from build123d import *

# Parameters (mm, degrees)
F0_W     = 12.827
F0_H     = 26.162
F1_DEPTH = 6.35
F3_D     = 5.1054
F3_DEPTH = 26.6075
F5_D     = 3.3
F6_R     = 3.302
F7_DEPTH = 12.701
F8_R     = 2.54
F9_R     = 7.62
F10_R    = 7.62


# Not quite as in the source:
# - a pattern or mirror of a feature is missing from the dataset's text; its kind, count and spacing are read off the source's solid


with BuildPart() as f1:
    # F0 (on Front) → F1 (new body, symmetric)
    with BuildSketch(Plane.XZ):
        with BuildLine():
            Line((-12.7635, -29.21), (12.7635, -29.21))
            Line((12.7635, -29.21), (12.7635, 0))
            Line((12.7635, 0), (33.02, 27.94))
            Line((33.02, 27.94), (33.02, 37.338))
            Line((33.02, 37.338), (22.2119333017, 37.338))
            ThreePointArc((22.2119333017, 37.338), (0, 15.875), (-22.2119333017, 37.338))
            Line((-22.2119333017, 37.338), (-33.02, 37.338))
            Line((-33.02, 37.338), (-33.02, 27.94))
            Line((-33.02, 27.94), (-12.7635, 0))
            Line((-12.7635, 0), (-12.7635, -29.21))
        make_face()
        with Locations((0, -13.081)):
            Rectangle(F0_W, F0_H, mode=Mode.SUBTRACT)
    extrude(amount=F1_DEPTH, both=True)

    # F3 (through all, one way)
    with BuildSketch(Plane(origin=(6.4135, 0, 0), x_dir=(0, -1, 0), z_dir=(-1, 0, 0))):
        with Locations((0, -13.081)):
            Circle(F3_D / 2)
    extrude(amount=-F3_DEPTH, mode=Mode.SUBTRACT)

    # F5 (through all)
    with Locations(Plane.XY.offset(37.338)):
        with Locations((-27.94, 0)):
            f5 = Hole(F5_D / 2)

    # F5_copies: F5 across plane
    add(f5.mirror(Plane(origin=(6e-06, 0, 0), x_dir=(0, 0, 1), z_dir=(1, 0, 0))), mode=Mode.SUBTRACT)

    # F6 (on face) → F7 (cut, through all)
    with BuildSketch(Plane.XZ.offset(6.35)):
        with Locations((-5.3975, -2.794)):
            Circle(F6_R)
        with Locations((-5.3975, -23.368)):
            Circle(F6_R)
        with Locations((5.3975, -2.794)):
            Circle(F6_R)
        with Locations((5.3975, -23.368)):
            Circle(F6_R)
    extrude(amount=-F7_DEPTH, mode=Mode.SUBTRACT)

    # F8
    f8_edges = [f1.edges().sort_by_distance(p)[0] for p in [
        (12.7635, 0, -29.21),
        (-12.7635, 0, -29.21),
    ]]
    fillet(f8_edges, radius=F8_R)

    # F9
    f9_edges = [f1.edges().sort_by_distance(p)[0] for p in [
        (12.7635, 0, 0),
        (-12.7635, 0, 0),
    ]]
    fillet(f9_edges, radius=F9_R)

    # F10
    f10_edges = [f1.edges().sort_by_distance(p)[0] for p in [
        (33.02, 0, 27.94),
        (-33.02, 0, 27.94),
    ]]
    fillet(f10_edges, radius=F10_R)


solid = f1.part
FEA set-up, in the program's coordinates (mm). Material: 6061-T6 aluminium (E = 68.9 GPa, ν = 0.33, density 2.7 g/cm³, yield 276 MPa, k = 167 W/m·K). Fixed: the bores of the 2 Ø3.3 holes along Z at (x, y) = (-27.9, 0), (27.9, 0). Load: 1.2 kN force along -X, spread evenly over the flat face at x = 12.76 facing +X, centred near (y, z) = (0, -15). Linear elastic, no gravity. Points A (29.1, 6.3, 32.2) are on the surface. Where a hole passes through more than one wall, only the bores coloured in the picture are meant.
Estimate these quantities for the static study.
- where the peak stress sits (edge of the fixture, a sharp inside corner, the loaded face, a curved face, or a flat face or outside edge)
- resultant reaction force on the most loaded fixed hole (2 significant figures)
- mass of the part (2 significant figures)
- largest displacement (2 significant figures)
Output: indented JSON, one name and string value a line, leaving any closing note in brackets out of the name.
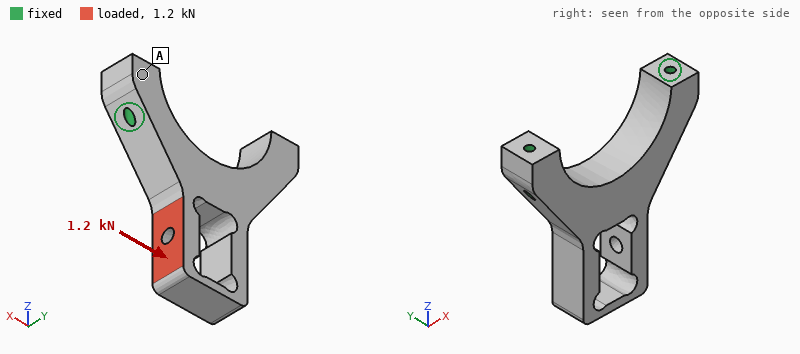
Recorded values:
{
  "where the peak stress sits": "a curved face",
  "resultant reaction force on the most loaded fixed hole": "1.2 kN",
  "mass of the part": "51 g",
  "largest displacement": "0.16 mm"
}
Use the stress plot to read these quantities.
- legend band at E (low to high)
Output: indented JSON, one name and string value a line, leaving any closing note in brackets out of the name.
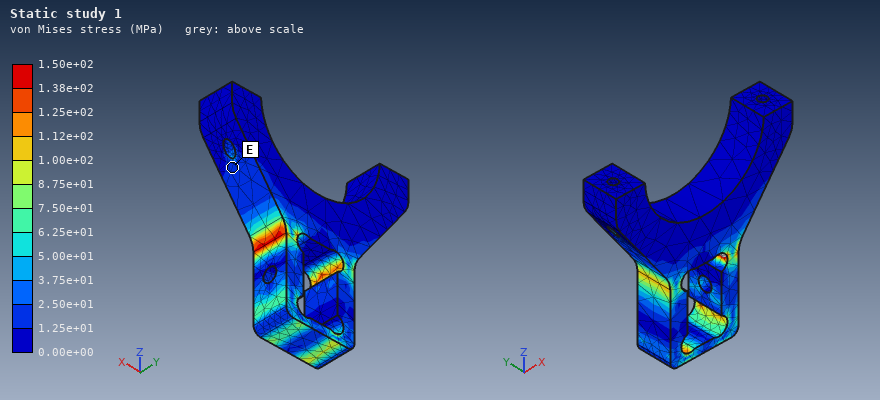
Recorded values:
{
  "legend band at E": "1.25e+01 to 2.50e+01 MPa"
}
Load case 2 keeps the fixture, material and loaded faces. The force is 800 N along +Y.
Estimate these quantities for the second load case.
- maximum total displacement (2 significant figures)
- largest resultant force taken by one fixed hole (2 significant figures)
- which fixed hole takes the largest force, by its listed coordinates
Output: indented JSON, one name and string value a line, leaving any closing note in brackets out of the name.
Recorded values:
{
  "maximum total displacement": "0.24 mm",
  "largest resultant force taken by one fixed hole": "600 N",
  "which fixed hole takes the largest force, by its listed coordinates": "(27.9, 0)"
}
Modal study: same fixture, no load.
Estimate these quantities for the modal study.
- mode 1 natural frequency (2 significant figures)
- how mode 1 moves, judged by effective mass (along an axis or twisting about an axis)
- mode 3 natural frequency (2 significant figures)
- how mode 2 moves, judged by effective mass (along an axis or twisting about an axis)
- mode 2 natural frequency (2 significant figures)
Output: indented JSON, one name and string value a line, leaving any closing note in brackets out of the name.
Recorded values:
{
  "mode 1 natural frequency": "3100 Hz",
  "how mode 1 moves, judged by effective mass": "along Y",
  "mode 3 natural frequency": "8200 Hz",
  "how mode 2 moves, judged by effective mass": "along X",
  "mode 2 natural frequency": "4300 Hz"
}
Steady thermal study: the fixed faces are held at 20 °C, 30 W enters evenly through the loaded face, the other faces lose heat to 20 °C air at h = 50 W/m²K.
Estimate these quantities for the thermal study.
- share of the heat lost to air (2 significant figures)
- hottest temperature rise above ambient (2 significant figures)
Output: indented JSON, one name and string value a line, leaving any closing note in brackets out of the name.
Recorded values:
{
  "share of the heat lost to air": "17 %",
  "hottest temperature rise above ambient": "48 K"
}
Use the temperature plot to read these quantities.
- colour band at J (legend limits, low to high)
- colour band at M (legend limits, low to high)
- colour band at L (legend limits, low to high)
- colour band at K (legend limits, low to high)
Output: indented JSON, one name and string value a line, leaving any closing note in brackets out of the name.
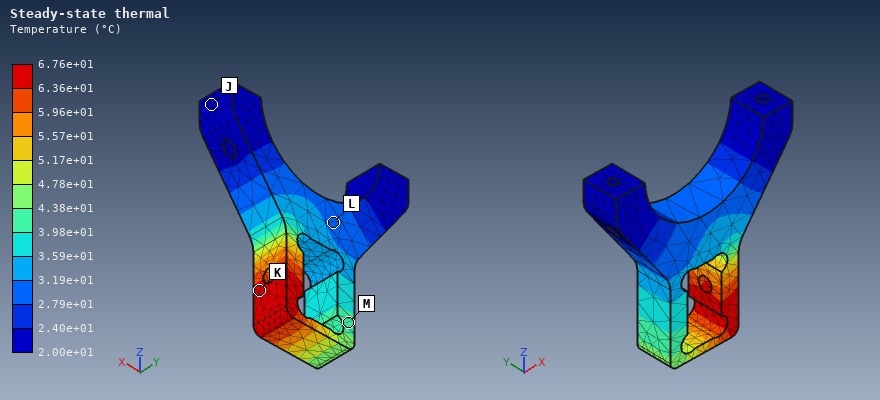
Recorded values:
{
  "colour band at J": "2.00e+01 to 2.40e+01 °C",
  "colour band at M": "3.98e+01 to 4.38e+01 °C",
  "colour band at L": "2.79e+01 to 3.19e+01 °C",
  "colour band at K": "6.36e+01 to 6.76e+01 °C"
}
